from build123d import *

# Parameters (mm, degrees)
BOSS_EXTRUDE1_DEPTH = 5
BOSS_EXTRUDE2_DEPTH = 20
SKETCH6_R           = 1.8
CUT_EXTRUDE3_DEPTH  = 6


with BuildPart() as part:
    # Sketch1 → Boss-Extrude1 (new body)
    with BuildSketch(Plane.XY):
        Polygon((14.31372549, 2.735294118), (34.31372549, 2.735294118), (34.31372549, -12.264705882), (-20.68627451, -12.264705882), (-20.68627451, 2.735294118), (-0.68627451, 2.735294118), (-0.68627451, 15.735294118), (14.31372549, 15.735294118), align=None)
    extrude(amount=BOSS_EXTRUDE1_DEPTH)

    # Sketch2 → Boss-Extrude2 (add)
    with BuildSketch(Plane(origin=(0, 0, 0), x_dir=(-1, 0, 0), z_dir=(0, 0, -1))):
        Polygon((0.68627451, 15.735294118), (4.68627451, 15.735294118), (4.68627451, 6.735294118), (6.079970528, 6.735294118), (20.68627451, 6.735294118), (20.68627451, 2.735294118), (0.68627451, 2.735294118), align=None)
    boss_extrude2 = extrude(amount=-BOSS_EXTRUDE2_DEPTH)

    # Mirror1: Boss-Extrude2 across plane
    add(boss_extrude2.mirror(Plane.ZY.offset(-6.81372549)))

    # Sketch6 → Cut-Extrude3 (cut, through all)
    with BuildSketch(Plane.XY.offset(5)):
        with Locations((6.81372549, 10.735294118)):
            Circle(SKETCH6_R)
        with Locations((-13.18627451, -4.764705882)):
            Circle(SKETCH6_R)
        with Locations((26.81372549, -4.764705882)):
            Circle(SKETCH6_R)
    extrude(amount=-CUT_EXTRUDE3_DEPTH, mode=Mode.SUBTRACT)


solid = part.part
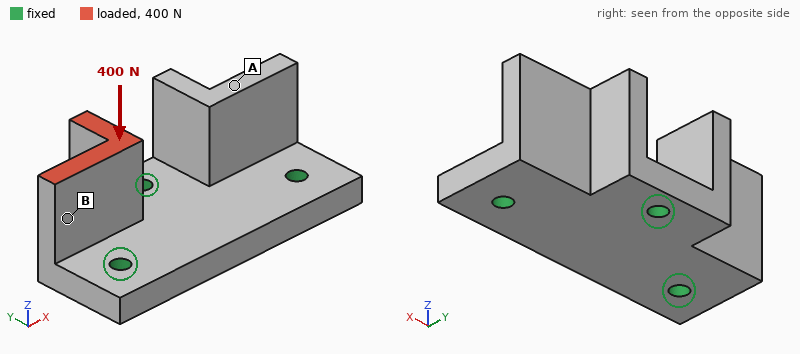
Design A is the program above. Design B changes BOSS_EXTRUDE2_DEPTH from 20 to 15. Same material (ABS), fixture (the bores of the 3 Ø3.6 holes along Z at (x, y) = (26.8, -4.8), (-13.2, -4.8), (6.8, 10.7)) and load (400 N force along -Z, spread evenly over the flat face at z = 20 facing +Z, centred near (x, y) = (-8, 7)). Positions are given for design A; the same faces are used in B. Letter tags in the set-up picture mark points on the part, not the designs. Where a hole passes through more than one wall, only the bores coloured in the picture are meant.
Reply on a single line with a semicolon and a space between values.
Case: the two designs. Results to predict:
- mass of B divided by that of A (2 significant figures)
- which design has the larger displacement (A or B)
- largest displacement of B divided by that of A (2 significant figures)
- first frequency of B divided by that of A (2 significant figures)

0.88; A; 0.92; 1.4
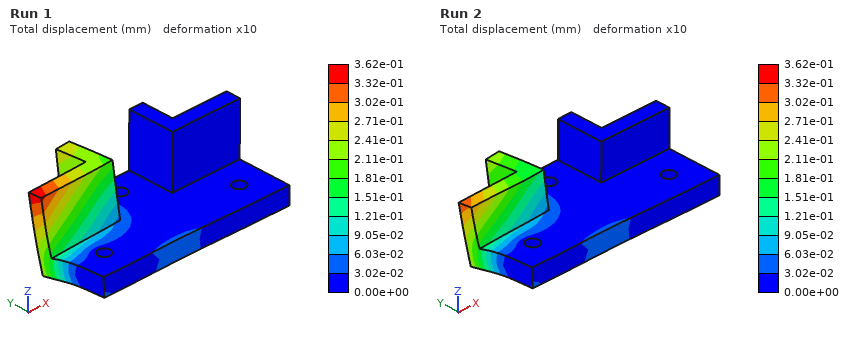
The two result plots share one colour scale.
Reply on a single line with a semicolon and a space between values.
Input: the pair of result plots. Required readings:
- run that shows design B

Run 2
